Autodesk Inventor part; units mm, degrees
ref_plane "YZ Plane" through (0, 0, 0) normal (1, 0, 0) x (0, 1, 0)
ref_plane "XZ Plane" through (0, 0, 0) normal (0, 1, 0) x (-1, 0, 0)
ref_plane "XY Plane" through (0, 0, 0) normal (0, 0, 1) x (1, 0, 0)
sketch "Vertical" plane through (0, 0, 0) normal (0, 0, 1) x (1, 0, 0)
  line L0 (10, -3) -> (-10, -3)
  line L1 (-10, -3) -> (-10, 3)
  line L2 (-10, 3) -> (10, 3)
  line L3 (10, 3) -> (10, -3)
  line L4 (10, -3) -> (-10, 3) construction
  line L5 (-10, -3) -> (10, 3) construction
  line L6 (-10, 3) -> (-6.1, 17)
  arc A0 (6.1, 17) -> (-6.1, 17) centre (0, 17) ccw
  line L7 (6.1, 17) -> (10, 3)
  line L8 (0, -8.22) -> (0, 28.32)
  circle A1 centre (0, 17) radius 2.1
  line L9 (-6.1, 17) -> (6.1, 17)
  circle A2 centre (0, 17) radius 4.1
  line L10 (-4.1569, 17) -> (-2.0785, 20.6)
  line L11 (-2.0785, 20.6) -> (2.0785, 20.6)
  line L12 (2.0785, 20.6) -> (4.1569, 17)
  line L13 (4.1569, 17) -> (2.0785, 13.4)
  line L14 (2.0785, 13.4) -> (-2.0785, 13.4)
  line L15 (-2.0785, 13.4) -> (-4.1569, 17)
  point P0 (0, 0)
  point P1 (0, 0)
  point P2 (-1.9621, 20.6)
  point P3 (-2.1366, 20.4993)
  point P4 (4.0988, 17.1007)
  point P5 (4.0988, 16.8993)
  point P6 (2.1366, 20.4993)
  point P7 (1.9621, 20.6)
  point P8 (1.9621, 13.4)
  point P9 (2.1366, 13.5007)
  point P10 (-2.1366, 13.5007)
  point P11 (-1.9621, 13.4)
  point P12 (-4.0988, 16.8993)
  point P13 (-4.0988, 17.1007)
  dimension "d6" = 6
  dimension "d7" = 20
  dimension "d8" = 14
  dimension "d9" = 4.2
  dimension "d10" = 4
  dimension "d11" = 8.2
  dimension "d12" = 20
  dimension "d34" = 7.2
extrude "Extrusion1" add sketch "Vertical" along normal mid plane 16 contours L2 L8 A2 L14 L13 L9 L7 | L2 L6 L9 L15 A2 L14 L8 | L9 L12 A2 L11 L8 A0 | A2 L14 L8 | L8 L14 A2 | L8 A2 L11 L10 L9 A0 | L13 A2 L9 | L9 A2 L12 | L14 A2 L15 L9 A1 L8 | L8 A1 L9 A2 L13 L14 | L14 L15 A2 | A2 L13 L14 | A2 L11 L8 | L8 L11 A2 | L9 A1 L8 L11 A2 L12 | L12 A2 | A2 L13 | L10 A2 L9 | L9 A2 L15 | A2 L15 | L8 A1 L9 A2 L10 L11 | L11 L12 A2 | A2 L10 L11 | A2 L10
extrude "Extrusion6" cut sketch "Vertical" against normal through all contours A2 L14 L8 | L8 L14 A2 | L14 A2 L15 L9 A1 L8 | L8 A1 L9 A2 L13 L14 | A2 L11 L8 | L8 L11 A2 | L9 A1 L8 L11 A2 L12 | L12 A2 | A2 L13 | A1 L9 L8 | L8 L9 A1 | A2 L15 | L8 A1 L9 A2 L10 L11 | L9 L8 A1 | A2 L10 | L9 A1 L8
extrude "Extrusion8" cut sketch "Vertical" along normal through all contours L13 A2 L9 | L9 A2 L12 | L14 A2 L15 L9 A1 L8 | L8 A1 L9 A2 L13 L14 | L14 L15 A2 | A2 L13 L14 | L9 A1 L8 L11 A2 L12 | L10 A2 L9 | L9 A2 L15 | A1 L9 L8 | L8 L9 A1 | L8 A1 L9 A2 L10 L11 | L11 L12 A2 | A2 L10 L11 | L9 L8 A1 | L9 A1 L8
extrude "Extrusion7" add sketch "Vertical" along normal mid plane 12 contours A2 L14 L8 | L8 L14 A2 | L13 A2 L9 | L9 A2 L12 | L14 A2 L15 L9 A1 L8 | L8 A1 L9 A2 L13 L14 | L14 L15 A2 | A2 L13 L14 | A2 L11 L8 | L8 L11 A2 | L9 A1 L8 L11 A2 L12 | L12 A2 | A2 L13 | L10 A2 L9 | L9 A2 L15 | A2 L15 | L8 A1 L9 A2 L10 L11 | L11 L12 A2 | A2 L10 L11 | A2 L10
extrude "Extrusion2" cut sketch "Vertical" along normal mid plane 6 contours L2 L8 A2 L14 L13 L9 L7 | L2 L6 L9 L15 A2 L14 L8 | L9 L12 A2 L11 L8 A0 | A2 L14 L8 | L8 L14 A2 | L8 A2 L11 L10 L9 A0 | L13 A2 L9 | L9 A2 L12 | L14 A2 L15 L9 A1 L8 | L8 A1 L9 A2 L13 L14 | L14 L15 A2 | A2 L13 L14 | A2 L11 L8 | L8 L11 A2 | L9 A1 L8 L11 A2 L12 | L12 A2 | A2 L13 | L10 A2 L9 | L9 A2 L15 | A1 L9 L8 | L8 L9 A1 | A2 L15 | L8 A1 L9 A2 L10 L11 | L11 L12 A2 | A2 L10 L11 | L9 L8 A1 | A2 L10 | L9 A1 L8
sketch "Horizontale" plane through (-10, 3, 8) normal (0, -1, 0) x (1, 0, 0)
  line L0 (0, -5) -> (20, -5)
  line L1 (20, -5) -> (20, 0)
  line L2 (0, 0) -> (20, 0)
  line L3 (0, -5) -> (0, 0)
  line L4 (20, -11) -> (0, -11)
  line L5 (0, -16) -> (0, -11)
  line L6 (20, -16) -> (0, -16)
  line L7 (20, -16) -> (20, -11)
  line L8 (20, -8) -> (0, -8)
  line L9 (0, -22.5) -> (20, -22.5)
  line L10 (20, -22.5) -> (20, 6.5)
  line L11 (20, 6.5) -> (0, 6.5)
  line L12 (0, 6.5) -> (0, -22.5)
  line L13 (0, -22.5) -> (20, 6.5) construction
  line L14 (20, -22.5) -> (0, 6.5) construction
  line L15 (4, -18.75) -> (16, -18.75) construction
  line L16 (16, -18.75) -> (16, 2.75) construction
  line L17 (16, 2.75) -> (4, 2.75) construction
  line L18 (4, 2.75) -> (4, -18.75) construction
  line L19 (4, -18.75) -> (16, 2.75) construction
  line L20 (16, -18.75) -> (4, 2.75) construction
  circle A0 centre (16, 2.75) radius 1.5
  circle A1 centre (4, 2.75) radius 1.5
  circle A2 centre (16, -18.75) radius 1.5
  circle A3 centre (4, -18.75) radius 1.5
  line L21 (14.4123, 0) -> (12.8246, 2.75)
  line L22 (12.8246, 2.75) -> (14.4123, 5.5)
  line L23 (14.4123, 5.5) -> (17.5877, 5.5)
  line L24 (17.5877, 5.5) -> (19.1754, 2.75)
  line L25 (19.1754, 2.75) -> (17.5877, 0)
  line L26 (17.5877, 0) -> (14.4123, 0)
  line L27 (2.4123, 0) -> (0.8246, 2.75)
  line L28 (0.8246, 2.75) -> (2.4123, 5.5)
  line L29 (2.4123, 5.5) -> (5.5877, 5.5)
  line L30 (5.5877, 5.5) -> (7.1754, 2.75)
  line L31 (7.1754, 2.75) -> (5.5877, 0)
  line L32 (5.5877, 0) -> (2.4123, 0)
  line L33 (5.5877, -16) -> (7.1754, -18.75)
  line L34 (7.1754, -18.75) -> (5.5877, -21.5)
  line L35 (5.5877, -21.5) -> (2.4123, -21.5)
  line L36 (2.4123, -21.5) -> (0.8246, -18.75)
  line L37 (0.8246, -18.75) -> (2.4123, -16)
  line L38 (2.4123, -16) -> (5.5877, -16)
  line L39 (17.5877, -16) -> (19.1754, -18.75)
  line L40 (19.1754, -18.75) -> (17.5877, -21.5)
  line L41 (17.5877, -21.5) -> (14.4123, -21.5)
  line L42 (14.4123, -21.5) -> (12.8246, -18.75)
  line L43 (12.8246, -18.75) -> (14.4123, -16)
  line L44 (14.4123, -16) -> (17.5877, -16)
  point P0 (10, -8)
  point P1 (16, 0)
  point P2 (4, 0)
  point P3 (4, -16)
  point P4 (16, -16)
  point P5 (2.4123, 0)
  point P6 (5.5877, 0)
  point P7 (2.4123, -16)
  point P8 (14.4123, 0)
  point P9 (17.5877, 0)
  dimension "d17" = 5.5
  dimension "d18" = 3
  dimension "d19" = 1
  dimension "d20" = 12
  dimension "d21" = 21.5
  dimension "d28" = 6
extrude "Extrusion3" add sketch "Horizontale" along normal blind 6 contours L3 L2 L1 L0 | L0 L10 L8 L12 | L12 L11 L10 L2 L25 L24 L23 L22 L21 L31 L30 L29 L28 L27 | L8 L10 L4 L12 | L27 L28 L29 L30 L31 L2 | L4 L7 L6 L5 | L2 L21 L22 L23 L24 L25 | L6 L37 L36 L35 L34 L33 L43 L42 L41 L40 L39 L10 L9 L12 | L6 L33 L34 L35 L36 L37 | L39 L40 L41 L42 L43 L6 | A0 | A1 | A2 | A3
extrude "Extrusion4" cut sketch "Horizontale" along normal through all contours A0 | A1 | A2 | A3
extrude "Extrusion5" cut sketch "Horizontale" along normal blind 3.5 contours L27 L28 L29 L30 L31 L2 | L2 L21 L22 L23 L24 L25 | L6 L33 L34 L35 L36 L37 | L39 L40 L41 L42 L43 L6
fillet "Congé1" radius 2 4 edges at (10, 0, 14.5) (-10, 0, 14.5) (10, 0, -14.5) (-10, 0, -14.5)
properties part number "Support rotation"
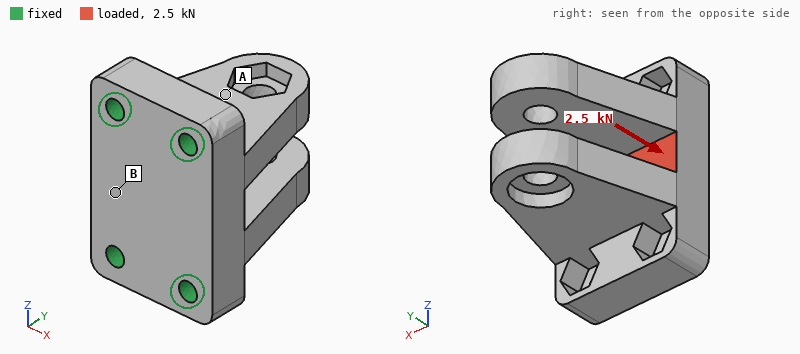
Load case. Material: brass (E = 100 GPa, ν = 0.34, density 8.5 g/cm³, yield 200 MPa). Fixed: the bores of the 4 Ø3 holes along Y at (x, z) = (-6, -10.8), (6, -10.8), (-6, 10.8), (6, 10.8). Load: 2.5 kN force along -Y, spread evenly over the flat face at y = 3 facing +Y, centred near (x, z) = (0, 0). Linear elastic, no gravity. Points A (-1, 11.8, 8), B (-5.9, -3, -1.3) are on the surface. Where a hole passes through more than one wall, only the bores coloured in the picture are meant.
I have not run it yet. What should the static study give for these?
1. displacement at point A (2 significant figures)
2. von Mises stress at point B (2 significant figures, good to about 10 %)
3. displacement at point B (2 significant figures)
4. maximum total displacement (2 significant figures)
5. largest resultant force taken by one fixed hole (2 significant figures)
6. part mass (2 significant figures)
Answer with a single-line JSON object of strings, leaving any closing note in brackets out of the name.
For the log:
{"displacement at point A": "10 µm", "von Mises stress at point B": "40 MPa", "displacement at point B": "8.4 µm", "maximum total displacement": "21 µm", "largest resultant force taken by one fixed hole": "810 N", "part mass": "47 g"}
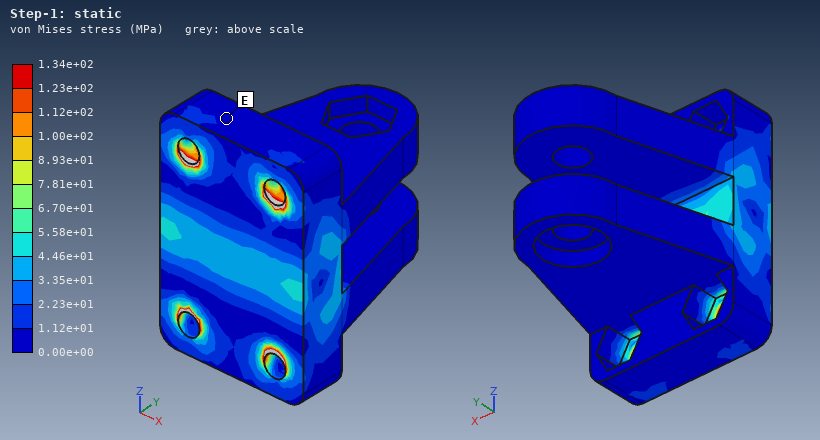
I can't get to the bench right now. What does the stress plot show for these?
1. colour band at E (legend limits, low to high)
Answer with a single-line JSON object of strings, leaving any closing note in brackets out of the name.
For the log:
{"colour band at E": "0.00e+00 to 1.12e+01 MPa"}
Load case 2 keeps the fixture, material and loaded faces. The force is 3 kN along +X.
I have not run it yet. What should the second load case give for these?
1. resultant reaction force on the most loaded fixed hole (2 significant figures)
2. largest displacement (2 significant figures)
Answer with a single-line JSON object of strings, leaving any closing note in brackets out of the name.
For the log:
{"resultant reaction force on the most loaded fixed hole": "1.0 kN", "largest displacement": "14 µm"}
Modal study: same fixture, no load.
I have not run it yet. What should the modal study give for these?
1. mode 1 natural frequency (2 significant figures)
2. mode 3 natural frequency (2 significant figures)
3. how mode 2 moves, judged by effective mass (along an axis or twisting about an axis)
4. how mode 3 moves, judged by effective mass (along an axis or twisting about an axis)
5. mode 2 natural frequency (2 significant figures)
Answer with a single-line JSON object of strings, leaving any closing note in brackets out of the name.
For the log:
{"mode 1 natural frequency": "7100 Hz", "mode 3 natural frequency": "10 kHz", "how mode 2 moves, judged by effective mass": "along Z", "how mode 3 moves, judged by effective mass": "along X", "mode 2 natural frequency": "7900 Hz"}
